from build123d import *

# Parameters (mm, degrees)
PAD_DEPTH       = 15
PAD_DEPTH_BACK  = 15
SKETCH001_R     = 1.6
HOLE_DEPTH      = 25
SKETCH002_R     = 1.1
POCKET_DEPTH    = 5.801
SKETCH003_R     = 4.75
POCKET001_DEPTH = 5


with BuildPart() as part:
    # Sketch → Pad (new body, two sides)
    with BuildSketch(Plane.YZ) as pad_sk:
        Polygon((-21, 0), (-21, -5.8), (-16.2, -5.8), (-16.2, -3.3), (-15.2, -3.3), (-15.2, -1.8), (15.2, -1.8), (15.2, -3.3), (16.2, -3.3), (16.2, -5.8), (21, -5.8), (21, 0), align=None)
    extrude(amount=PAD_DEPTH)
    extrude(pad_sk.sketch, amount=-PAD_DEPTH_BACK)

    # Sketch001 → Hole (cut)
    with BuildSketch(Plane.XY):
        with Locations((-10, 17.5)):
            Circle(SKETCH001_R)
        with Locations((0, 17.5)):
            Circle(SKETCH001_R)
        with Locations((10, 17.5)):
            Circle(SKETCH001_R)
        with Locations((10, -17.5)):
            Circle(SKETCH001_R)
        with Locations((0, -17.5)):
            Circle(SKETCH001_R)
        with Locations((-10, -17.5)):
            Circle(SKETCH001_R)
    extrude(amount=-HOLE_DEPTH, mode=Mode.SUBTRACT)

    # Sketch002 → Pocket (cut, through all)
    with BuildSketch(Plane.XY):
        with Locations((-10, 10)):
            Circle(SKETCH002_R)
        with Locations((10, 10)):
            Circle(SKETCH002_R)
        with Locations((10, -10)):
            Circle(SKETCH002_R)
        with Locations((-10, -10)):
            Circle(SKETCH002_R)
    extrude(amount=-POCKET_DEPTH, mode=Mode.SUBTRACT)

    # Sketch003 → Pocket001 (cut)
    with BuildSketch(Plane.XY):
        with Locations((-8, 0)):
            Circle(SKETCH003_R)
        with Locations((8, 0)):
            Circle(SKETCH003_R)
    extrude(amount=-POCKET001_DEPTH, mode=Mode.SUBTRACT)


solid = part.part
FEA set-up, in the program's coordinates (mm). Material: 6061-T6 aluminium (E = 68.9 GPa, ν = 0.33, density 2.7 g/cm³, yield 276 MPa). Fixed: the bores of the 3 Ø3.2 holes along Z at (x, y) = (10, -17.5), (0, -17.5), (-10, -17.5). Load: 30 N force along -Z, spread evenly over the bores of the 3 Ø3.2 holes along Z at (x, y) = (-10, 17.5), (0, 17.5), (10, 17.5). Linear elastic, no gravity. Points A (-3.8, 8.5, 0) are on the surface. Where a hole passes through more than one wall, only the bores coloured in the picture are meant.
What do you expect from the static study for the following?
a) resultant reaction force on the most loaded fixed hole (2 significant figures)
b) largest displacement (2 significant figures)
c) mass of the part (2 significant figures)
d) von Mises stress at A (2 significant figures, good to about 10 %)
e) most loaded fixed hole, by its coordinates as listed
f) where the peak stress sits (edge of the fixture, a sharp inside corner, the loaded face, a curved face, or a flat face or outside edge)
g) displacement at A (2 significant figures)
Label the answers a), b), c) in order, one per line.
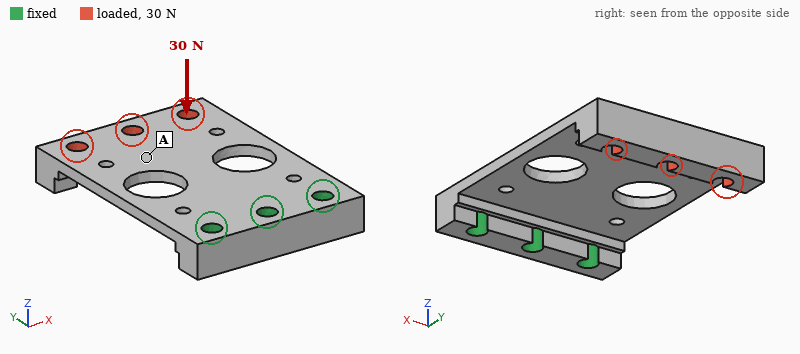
a) 18 N
b) 0.60 mm
c) 8.0 g
d) 18 MPa
e) (0, -17.5)
f) a curved face
g) 0.29 mm
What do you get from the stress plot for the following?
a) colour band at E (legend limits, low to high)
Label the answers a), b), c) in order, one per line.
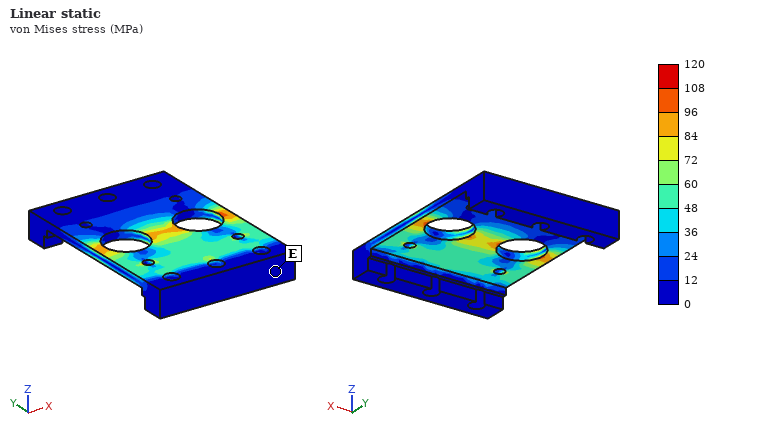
a) 0 to 12 MPa
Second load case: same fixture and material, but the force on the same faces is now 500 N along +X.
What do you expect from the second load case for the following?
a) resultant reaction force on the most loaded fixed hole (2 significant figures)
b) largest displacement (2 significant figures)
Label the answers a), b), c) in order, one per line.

a) 790 N
b) 0.30 mm
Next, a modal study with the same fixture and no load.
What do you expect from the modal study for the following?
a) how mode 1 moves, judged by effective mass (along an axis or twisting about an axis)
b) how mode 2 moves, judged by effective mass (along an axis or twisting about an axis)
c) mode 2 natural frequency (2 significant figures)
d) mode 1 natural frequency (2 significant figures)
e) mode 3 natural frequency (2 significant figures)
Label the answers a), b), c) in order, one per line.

a) along Z
b) twisting about Y
c) 2300 Hz
d) 700 Hz
e) 5500 Hz
